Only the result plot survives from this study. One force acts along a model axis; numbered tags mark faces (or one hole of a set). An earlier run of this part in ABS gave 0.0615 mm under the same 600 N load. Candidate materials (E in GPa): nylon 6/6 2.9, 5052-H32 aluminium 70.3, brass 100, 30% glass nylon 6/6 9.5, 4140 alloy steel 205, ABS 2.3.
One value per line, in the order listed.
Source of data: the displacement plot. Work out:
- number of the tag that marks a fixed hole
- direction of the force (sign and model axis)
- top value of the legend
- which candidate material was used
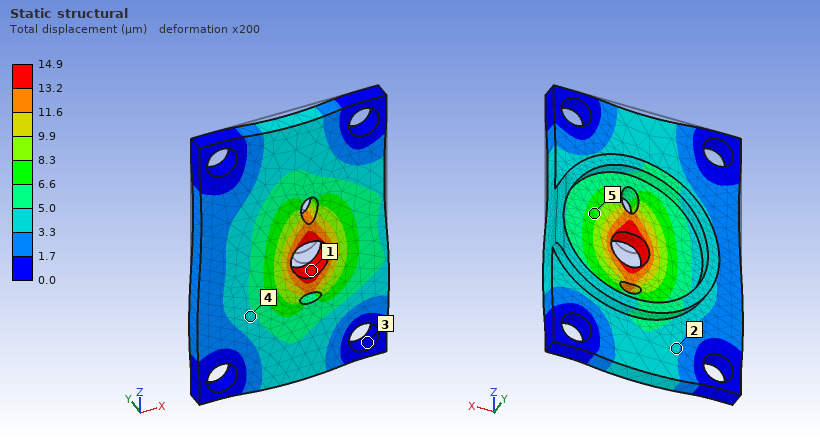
3
-Z
14.9 µm
30% glass nylon 6/6
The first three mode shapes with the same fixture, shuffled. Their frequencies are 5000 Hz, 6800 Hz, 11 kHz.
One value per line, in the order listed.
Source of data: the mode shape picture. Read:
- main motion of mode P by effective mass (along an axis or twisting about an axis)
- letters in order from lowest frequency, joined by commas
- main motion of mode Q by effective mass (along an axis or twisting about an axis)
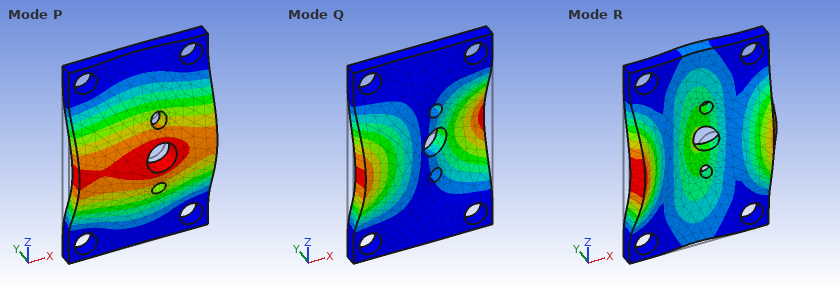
along Y
P, Q, R
twisting about Z
